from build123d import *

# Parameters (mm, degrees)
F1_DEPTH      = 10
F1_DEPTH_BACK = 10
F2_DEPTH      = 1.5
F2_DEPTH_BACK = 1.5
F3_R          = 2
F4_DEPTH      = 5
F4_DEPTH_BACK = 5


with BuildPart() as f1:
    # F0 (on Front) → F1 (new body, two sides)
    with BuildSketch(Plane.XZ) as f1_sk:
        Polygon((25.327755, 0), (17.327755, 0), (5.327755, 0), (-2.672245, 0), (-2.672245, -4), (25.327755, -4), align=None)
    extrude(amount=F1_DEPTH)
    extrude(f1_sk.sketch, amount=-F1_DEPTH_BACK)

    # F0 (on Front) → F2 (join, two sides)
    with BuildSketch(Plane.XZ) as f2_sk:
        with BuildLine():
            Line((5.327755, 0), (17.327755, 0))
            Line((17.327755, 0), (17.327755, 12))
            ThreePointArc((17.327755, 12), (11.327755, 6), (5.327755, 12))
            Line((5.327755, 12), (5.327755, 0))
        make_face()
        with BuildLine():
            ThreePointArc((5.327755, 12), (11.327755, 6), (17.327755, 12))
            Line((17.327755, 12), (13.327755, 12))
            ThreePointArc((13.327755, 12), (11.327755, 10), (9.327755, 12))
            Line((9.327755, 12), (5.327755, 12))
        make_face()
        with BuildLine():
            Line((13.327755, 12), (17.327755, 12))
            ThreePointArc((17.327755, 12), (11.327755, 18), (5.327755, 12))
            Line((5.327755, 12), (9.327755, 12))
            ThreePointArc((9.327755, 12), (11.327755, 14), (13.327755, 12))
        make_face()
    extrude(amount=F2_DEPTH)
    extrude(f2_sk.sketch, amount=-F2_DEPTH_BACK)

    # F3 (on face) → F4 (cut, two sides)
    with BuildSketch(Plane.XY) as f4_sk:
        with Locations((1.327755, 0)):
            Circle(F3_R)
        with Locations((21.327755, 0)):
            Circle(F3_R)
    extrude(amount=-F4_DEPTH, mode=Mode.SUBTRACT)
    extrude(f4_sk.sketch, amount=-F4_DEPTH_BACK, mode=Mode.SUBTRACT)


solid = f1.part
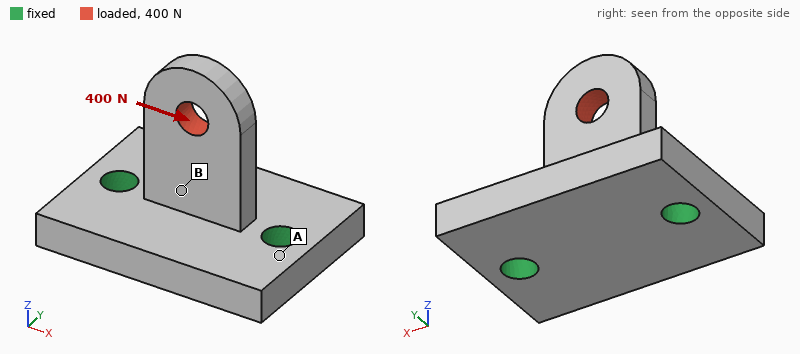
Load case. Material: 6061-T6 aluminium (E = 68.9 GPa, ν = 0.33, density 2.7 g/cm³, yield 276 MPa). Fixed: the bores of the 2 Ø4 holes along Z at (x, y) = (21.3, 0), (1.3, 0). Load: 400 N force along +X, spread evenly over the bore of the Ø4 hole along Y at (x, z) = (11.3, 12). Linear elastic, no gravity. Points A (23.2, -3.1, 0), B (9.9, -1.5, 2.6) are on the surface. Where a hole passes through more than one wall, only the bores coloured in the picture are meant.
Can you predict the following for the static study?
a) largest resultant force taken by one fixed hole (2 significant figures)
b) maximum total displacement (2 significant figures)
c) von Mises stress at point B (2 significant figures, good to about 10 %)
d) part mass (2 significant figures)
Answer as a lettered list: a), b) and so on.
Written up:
a) 420 N
b) 30 µm
c) 24 MPa
d) 7.3 g
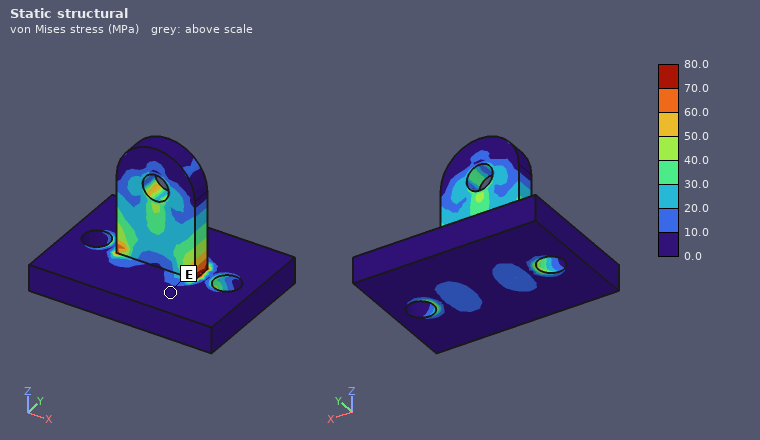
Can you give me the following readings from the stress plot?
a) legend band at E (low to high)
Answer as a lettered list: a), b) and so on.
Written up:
a) 0.0 to 10.0 MPa
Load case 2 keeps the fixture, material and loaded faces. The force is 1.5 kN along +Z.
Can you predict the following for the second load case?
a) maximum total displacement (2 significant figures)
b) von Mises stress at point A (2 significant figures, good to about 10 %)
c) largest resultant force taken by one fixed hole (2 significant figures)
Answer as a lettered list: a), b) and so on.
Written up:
a) 18 µm
b) 13 MPa
c) 770 N
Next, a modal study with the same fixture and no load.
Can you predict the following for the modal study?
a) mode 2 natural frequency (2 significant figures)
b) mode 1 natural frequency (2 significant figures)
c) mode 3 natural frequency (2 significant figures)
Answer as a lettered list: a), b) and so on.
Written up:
a) 22 kHz
b) 7600 Hz
c) 24 kHz
